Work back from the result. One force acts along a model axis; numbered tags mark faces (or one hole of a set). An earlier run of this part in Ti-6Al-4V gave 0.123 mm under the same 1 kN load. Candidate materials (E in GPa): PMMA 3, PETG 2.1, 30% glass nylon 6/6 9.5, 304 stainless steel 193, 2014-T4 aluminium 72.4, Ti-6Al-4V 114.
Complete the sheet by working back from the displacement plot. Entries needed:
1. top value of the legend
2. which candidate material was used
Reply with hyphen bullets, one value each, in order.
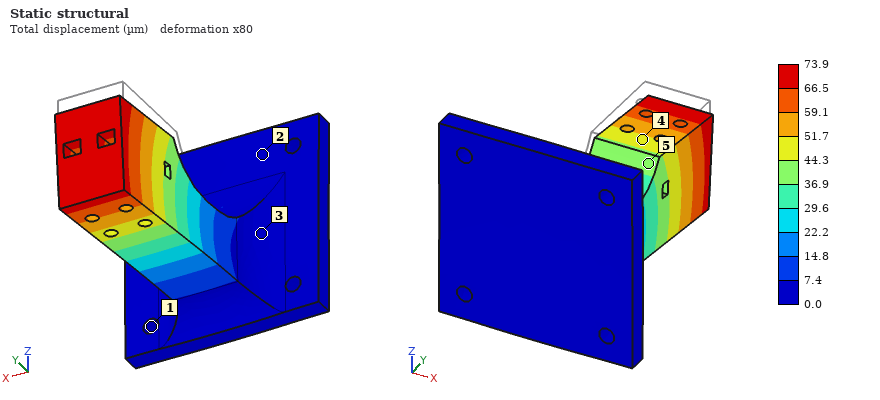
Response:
- 73.9 µm
- 304 stainless steel
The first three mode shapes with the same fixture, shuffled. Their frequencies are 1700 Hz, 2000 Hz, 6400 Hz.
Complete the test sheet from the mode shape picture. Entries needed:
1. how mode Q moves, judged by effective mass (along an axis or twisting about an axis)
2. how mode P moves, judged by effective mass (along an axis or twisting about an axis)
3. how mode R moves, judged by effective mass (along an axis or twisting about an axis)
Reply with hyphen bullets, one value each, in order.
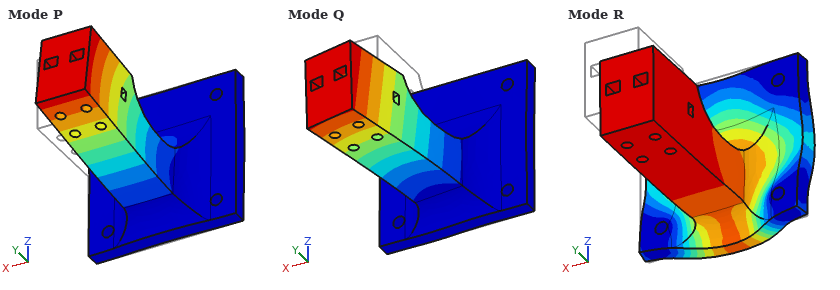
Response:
- along X
- along Z
- along Y
